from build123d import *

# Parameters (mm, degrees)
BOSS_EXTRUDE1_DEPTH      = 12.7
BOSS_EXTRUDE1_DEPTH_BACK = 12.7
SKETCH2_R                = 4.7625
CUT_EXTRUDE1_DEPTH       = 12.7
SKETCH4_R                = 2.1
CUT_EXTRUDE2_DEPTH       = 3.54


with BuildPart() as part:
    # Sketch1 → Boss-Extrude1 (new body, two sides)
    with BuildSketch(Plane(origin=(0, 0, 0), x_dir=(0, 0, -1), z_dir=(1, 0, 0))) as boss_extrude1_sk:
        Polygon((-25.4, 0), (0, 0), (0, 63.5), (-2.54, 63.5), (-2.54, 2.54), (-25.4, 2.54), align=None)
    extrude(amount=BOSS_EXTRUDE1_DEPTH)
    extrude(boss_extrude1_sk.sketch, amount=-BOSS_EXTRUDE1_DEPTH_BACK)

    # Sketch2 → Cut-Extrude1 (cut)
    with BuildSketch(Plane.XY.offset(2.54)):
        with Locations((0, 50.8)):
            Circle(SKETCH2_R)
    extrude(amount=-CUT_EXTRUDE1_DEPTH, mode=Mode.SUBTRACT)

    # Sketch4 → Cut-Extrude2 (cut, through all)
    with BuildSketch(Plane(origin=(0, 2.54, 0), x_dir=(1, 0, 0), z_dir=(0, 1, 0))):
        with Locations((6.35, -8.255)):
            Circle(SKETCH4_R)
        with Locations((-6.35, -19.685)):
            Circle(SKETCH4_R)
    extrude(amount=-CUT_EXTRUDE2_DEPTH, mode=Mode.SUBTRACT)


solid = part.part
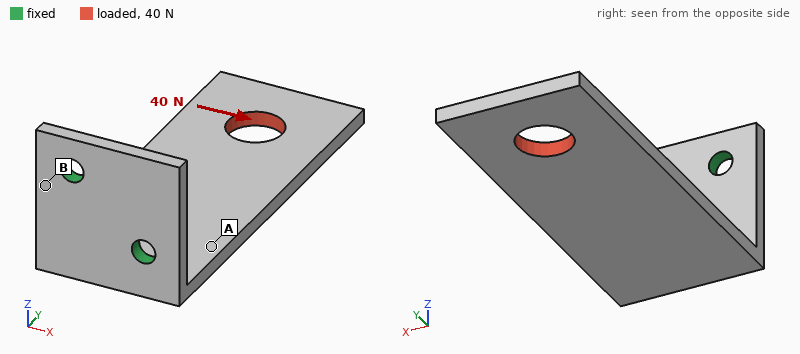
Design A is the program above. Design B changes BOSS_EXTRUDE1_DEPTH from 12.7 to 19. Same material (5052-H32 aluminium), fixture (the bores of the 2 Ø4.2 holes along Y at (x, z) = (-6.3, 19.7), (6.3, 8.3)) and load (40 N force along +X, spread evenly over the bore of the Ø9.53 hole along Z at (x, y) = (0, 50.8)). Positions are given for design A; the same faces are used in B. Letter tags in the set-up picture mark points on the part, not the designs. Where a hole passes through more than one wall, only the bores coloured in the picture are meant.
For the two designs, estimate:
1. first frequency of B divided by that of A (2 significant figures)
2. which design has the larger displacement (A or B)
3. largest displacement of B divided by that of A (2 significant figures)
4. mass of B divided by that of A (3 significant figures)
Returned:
1.00
A
0.76
1.26
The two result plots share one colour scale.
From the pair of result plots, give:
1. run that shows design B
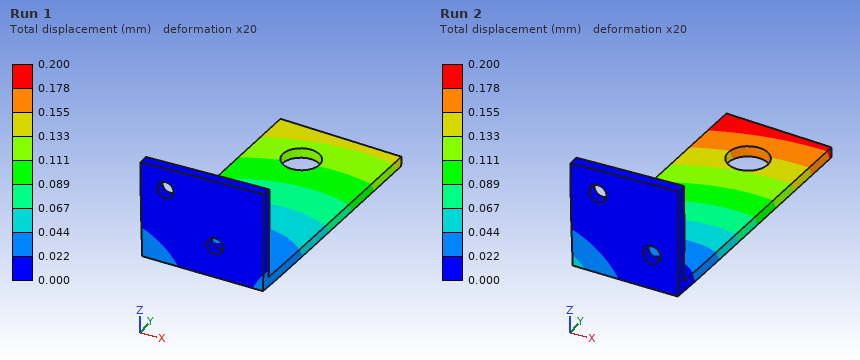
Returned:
Run 1
